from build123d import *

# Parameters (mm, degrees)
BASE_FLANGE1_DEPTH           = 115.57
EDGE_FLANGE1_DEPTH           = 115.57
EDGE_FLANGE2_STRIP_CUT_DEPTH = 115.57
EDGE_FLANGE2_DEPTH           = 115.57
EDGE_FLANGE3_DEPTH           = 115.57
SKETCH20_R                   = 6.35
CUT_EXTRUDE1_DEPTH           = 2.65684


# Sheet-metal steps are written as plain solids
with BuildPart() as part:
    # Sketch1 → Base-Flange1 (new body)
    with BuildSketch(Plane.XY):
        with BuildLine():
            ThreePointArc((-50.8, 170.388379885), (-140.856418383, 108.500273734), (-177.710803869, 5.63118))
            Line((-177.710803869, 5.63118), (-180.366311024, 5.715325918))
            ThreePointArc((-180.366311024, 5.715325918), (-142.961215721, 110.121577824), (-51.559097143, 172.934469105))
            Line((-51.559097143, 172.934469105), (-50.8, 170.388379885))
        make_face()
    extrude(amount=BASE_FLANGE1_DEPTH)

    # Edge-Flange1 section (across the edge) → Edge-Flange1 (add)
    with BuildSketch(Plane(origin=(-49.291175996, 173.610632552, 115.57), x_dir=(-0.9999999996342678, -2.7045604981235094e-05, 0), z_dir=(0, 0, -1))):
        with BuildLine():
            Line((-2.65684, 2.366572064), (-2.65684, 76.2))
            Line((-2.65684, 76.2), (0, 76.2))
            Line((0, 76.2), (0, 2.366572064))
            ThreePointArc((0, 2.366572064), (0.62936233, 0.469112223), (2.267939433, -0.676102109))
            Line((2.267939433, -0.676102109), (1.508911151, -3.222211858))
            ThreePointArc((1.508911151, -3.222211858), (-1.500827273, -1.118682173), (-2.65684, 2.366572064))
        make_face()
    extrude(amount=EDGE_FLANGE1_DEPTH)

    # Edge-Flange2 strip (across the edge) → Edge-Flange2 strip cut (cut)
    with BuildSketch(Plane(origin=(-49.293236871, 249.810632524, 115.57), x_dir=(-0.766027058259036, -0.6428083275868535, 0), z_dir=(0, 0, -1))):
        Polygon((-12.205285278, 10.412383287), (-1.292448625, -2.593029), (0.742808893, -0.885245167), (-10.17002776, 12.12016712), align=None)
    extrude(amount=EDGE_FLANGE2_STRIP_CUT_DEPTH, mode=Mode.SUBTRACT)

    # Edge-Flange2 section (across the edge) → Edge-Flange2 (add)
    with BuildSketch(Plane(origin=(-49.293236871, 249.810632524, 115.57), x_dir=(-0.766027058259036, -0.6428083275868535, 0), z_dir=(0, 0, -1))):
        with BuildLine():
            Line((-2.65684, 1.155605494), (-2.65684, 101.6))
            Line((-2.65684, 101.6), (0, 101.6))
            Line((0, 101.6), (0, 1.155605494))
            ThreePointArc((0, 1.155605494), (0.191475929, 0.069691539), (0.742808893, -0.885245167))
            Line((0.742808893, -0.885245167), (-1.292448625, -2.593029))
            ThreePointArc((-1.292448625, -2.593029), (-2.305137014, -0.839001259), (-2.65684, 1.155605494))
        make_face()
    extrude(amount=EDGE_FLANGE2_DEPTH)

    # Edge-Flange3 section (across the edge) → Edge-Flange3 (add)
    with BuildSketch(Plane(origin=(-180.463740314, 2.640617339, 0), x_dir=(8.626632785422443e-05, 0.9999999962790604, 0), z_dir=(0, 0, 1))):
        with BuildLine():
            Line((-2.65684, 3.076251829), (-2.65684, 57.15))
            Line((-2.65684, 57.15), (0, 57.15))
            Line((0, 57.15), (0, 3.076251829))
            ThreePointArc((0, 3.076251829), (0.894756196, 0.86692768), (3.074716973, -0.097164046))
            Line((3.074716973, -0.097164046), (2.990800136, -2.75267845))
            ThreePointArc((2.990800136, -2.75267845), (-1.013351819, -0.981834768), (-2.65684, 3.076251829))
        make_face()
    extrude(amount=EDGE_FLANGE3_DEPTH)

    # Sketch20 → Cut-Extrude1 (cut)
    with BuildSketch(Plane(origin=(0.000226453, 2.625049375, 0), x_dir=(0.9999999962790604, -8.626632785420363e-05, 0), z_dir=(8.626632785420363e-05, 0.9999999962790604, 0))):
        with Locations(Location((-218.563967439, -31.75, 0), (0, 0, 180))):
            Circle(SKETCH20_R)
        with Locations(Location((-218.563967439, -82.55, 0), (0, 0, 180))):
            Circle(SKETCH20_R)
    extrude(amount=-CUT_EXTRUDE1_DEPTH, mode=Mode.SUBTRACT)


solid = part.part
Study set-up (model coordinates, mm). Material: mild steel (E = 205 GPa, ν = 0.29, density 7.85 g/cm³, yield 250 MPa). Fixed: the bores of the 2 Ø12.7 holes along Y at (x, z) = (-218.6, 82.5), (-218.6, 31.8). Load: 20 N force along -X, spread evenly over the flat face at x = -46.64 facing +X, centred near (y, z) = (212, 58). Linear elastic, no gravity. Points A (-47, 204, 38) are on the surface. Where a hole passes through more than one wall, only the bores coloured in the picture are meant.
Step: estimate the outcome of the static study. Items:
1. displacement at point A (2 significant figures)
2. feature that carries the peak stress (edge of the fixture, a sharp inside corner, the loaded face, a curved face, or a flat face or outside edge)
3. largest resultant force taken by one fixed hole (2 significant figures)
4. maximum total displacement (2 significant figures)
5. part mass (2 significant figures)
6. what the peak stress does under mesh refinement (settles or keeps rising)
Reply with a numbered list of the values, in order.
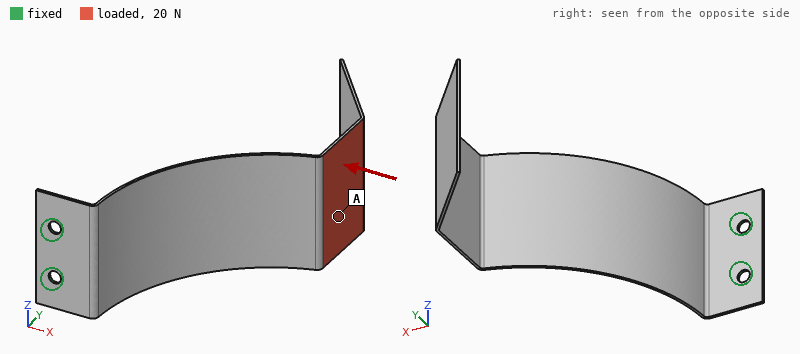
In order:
1. 3.1 mm
2. edge of the fixture
3. 12 N
4. 4.6 mm
5. 1.1 kg
6. keeps rising
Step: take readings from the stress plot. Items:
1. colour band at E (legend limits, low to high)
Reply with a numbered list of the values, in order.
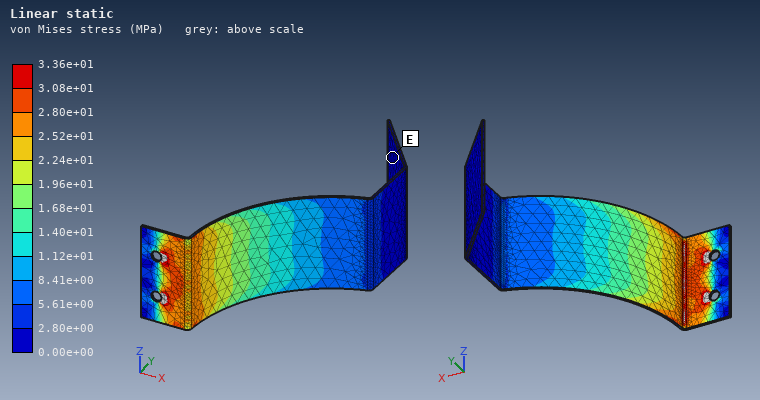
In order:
1. 0.00e+00 to 2.80e+00 MPa
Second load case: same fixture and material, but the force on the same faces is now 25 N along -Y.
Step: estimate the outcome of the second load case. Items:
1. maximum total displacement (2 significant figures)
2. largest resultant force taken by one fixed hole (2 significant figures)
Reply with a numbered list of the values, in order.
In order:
1. 4.3 mm
2. 14 N
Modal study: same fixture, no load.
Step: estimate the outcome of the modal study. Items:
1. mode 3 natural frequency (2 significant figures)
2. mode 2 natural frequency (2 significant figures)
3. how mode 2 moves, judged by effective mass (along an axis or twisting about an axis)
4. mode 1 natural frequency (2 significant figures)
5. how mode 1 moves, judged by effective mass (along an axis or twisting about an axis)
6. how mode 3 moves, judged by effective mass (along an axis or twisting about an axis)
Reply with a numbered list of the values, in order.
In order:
1. 66 Hz
2. 47 Hz
3. along Z
4. 13 Hz
5. along X
6. along Y
